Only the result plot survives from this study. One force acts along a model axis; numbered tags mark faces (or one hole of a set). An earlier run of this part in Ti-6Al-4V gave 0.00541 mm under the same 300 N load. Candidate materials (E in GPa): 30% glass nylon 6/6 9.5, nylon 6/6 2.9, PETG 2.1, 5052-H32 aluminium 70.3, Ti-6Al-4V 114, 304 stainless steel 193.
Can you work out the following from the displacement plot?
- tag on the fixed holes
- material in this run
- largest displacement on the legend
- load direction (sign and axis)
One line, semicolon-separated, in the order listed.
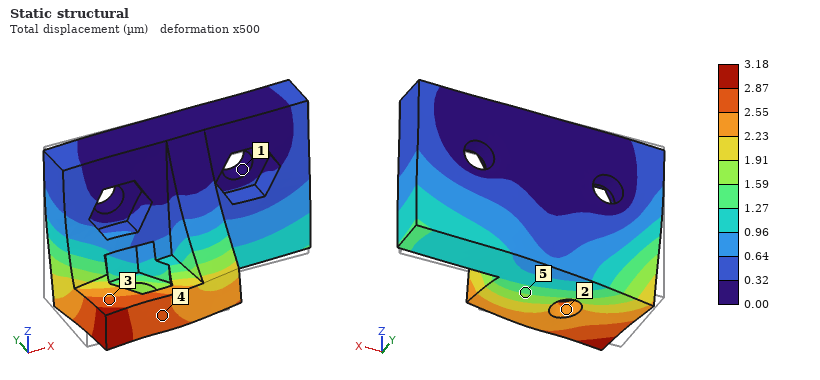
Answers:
1; 304 stainless steel; 3.18 µm; +X
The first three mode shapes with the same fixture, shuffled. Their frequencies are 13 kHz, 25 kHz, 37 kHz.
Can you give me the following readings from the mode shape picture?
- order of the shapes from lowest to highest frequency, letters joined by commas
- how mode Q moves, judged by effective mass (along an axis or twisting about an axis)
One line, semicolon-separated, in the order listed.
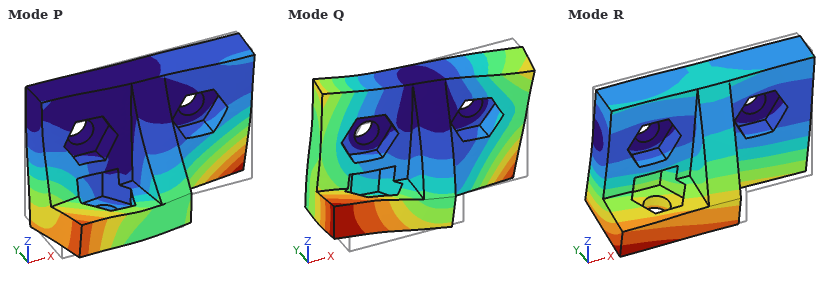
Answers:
R, P, Q; along X
